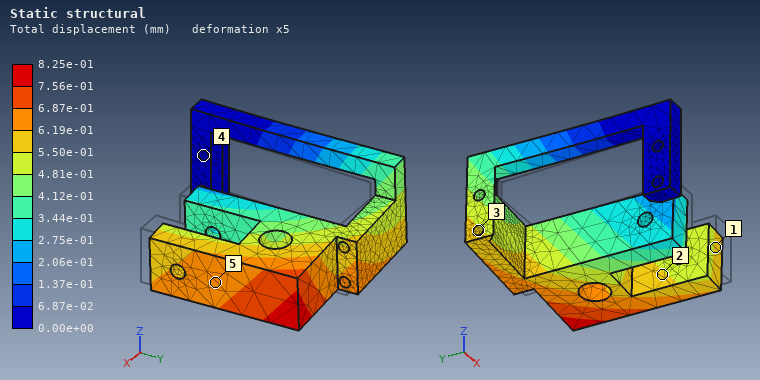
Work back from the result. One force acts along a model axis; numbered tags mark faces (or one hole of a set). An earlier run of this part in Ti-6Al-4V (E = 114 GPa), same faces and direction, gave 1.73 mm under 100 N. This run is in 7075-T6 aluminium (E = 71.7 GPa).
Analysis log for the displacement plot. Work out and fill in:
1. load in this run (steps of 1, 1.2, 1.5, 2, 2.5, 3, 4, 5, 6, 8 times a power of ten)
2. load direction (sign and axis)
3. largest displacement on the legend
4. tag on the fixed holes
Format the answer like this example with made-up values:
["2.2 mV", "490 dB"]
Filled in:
["30 N", "-X", "8.25e-01 mm", "4"]
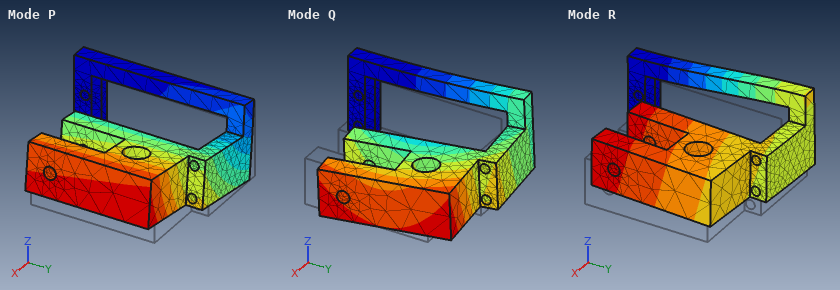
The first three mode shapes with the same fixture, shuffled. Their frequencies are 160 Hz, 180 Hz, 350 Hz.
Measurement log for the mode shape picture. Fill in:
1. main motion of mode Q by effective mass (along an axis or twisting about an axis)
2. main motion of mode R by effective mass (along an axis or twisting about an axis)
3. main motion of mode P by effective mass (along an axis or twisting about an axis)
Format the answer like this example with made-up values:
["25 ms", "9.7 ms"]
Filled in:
["along Y", "along X", "along Z"]
